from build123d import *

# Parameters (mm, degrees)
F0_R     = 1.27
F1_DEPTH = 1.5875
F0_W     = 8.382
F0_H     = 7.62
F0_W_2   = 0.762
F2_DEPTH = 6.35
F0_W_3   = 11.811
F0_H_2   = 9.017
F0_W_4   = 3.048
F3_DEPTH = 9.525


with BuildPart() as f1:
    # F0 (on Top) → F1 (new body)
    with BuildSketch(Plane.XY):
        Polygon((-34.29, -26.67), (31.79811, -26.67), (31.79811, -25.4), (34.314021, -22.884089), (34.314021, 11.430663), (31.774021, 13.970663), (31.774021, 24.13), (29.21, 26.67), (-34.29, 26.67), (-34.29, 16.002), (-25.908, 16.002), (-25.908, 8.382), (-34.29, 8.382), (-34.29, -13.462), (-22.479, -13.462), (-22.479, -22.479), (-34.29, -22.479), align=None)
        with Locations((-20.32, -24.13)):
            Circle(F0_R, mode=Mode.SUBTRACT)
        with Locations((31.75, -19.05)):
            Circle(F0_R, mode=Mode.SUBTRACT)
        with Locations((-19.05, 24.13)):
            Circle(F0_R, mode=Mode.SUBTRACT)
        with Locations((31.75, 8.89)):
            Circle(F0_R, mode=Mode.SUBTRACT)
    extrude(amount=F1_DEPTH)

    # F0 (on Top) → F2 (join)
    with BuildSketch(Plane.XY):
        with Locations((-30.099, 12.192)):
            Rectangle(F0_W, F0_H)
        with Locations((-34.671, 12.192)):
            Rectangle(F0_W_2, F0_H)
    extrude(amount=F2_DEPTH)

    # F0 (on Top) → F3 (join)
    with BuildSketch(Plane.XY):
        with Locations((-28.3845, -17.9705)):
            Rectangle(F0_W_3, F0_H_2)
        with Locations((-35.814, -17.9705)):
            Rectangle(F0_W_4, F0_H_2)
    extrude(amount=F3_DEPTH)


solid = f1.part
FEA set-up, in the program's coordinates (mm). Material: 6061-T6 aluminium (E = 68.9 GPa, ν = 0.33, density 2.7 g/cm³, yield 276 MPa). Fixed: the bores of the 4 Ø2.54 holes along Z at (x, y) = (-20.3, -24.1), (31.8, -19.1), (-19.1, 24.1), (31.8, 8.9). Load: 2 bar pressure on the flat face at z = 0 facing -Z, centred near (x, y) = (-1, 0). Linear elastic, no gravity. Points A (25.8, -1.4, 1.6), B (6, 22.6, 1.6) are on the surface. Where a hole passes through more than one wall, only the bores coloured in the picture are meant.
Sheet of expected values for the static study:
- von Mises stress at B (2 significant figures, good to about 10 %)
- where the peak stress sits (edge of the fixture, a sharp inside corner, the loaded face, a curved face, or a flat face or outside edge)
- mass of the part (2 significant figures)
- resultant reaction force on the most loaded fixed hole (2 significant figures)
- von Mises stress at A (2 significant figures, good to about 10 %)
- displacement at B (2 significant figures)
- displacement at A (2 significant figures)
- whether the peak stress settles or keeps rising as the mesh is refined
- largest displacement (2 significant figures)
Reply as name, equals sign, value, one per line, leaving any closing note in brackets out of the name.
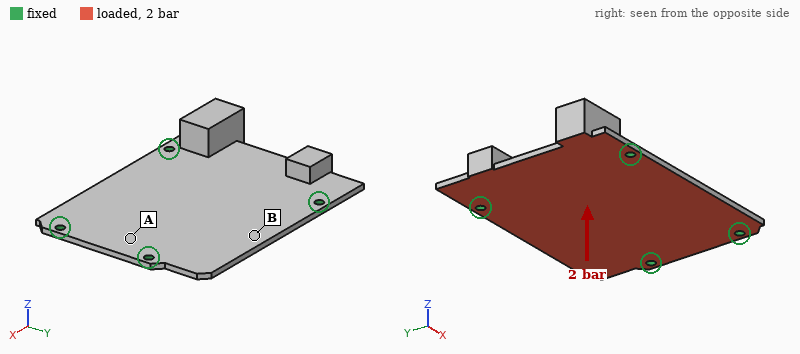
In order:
von Mises stress at B = 70 MPa
where the peak stress sits = edge of the fixture
mass of the part = 19 g
resultant reaction force on the most loaded fixed hole = 220 N
von Mises stress at A = 30 MPa
displacement at B = 0.25 mm
displacement at A = 0.066 mm
whether the peak stress settles or keeps rising as the mesh is refined = keeps rising
largest displacement = 0.27 mm
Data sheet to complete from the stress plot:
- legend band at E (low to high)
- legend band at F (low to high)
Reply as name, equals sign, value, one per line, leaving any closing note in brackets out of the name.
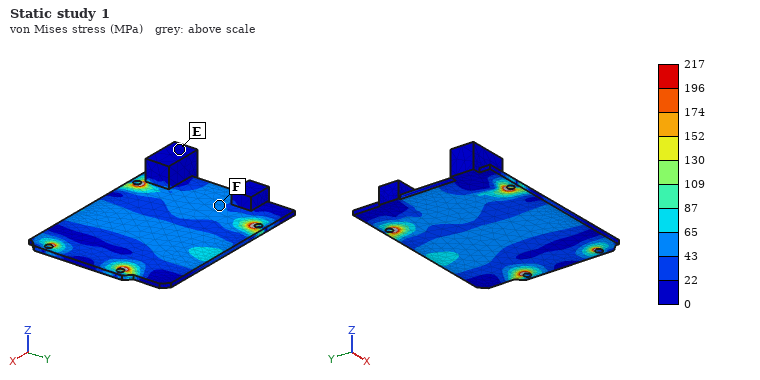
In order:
legend band at E = 0 to 22 MPa
legend band at F = 43 to 65 MPa
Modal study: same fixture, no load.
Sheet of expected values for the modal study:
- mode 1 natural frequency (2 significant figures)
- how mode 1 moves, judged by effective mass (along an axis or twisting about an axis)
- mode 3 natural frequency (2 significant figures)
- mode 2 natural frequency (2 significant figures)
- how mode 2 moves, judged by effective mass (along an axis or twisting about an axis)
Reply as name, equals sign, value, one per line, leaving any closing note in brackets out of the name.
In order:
mode 1 natural frequency = 2000 Hz
how mode 1 moves, judged by effective mass = along Z
mode 3 natural frequency = 3000 Hz
mode 2 natural frequency = 2400 Hz
how mode 2 moves, judged by effective mass = along Z
